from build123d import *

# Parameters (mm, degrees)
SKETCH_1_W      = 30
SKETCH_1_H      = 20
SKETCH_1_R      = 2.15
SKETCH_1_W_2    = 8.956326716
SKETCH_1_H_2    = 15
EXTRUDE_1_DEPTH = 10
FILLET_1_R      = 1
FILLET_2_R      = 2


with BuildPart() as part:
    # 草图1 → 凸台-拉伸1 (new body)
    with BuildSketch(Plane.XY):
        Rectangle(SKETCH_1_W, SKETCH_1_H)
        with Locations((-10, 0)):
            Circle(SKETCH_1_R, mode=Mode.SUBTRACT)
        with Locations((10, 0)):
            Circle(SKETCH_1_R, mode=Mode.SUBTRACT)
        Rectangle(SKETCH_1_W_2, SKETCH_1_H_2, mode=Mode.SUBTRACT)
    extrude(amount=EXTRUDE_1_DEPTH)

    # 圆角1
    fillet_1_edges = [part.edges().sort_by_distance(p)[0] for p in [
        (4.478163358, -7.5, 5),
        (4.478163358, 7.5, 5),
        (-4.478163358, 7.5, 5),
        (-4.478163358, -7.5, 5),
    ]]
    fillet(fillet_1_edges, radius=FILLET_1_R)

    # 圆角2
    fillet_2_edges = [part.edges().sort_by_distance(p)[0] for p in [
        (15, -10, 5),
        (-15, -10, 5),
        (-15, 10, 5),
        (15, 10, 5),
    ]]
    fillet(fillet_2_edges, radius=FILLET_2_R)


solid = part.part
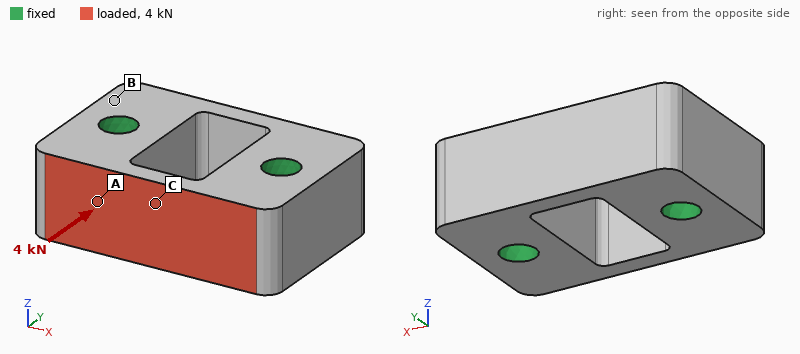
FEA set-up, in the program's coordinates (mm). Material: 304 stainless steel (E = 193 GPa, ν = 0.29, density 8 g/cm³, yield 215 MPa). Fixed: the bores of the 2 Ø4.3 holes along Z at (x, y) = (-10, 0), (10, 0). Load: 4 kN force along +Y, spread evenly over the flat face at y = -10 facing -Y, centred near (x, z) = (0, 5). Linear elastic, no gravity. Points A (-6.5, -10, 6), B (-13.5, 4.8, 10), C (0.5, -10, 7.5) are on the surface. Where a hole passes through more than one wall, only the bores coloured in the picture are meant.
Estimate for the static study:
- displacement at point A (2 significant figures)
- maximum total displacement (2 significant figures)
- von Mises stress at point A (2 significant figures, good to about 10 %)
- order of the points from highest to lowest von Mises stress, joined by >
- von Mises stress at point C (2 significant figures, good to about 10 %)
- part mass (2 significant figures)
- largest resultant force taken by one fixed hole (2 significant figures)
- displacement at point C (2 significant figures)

1.5 µm
4.9 µm
34 MPa
C > A > B
77 MPa
35 g
2.1 kN
4.5 µm
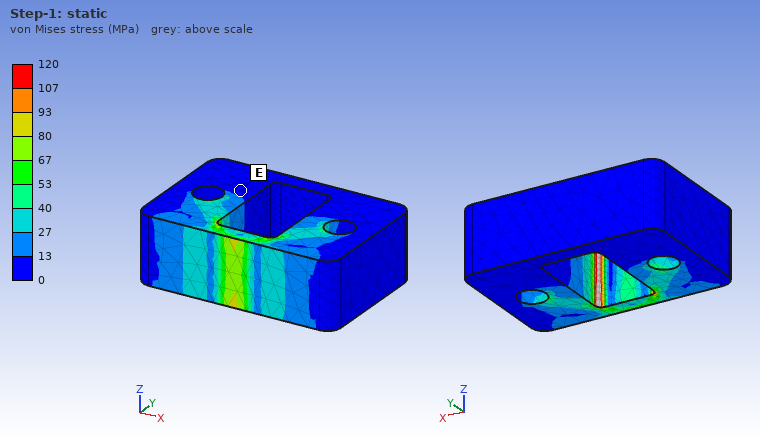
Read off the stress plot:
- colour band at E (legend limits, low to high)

0 to 13 MPa
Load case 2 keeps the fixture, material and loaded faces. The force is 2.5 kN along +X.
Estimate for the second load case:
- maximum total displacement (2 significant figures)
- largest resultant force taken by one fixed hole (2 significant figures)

4.1 µm
1.3 kN
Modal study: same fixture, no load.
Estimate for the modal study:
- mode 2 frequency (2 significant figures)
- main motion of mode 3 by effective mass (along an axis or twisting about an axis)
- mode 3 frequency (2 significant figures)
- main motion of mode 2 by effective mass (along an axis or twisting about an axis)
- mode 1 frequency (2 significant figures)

47 kHz
along Z
51 kHz
twisting about X
40 kHz
